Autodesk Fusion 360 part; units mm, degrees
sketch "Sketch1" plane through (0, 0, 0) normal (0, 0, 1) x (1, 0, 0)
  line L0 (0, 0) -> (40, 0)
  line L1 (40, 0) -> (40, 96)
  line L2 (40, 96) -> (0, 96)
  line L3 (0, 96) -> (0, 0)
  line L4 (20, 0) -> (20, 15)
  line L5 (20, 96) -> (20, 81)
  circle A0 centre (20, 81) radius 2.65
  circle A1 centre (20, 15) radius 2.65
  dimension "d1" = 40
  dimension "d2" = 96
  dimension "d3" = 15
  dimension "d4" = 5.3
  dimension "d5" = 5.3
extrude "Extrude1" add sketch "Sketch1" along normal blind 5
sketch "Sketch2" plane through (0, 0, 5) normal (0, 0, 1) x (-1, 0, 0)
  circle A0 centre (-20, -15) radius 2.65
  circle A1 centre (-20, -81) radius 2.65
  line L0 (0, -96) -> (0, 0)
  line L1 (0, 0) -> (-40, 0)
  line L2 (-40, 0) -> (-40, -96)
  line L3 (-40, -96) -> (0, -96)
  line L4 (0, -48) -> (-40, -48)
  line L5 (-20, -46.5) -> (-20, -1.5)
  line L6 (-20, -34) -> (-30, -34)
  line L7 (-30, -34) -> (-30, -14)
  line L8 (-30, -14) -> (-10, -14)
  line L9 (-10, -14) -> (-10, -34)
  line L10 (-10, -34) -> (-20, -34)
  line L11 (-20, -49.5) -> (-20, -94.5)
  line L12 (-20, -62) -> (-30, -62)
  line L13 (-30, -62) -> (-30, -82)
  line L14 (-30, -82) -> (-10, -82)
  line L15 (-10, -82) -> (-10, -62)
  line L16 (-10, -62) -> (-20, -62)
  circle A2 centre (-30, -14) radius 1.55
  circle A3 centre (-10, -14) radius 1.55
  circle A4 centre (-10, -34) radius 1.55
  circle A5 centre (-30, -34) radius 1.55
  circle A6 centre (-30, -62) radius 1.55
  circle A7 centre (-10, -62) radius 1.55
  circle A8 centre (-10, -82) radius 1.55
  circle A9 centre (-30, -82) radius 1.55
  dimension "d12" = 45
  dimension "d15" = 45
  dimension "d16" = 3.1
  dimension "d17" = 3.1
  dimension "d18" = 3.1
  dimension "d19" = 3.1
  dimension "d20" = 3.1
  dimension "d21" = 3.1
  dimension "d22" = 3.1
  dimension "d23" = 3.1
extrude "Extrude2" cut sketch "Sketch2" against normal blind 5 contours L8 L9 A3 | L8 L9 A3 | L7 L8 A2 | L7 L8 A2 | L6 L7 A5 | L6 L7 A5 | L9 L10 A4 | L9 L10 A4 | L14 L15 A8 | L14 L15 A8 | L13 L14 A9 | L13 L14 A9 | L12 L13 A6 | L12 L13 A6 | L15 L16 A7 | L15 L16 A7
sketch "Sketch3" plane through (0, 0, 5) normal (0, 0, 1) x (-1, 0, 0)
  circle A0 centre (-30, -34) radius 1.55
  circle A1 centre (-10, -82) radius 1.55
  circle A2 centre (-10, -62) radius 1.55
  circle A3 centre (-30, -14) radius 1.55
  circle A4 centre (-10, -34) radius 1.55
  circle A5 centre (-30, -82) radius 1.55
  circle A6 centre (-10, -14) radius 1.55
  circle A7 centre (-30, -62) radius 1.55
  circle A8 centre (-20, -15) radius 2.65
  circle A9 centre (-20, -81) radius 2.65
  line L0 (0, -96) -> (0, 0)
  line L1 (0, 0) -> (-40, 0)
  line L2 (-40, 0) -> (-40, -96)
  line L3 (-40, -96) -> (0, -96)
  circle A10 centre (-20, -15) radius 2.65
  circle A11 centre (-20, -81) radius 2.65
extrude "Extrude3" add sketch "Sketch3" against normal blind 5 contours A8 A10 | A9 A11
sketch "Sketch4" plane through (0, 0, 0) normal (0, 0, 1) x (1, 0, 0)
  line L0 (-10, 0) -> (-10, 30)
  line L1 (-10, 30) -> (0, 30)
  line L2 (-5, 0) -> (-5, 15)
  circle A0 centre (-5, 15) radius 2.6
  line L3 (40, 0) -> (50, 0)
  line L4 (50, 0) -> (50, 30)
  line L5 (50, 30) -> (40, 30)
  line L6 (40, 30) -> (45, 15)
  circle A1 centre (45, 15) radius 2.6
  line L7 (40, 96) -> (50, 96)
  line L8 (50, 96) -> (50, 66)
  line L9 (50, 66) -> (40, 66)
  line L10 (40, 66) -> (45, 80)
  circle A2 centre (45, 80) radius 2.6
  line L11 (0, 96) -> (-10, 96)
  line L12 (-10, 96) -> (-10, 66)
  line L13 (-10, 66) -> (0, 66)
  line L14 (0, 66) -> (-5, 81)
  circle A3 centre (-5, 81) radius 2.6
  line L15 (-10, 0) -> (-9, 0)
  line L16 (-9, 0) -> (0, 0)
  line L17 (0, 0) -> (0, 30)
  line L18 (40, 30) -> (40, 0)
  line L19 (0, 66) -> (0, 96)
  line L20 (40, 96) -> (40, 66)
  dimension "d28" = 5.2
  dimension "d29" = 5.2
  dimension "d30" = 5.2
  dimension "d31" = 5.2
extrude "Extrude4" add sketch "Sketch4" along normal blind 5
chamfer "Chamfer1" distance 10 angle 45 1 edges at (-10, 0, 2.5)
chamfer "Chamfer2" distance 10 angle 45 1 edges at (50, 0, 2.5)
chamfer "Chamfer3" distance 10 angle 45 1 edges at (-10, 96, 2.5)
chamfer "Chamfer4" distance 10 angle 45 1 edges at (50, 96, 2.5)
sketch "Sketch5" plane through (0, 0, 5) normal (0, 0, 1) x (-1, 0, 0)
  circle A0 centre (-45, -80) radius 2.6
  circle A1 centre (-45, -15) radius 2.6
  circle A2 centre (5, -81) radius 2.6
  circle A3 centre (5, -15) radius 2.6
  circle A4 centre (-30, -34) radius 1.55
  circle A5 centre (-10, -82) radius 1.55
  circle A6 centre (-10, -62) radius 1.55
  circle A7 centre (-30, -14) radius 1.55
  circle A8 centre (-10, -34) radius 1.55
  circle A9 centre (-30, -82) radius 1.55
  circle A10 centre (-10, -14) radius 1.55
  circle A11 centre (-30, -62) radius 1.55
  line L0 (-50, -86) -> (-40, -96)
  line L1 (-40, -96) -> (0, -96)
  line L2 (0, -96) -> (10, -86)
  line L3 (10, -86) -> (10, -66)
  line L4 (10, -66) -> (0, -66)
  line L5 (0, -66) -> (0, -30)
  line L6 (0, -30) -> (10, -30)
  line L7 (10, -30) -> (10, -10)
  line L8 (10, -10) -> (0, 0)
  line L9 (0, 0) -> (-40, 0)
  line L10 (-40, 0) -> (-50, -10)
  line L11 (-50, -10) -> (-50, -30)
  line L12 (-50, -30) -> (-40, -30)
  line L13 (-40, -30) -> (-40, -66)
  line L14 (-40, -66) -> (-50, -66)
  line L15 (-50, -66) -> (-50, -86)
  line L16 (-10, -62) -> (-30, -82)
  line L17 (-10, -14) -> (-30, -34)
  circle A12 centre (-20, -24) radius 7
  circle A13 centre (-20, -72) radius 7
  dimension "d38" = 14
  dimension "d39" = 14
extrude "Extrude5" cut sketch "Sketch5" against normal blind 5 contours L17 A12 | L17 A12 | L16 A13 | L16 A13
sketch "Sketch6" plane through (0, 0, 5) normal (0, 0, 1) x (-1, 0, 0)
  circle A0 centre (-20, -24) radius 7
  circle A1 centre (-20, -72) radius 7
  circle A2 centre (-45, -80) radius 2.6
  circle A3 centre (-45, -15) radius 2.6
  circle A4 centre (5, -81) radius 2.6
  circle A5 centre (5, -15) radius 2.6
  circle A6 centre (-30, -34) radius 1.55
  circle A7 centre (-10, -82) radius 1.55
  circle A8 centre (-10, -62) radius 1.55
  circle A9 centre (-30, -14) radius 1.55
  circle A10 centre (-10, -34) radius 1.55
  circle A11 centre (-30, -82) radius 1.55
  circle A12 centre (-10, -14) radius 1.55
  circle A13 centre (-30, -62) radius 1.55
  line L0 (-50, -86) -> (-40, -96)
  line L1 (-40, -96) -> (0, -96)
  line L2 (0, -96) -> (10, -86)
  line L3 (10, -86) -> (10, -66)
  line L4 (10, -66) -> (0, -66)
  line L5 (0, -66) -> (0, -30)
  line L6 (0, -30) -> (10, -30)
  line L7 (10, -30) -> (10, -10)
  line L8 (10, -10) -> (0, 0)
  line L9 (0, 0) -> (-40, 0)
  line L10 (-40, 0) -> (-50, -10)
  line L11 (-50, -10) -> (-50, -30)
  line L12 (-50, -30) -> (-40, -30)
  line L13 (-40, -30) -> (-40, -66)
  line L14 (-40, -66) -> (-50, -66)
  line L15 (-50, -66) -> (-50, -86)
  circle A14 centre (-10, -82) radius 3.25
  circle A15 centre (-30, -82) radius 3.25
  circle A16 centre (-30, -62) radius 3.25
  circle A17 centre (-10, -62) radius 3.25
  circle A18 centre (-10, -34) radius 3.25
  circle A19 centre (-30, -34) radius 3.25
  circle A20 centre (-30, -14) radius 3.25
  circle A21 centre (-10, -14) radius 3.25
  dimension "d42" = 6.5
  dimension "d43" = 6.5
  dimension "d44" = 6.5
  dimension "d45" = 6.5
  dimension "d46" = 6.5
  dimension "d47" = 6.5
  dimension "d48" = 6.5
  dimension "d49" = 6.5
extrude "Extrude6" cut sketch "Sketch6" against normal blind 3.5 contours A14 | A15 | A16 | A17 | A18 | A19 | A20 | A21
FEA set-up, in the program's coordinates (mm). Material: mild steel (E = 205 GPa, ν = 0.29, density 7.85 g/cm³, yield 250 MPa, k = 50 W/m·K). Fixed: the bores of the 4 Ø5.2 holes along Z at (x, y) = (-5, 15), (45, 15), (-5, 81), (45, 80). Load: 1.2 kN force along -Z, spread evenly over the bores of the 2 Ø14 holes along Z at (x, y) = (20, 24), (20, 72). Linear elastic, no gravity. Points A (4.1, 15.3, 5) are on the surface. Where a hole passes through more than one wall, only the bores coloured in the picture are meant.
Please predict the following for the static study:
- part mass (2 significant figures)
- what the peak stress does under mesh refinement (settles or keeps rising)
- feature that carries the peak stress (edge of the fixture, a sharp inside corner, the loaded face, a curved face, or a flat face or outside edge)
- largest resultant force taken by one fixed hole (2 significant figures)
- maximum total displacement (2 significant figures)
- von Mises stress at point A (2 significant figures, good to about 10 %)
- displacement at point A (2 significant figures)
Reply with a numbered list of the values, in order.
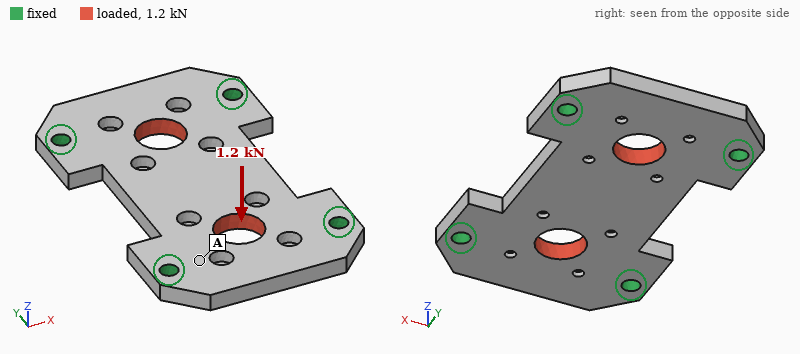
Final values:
1. 170 g
2. keeps rising
3. edge of the fixture
4. 310 N
5. 13 µm
6. 21 MPa
7. 2.6 µm
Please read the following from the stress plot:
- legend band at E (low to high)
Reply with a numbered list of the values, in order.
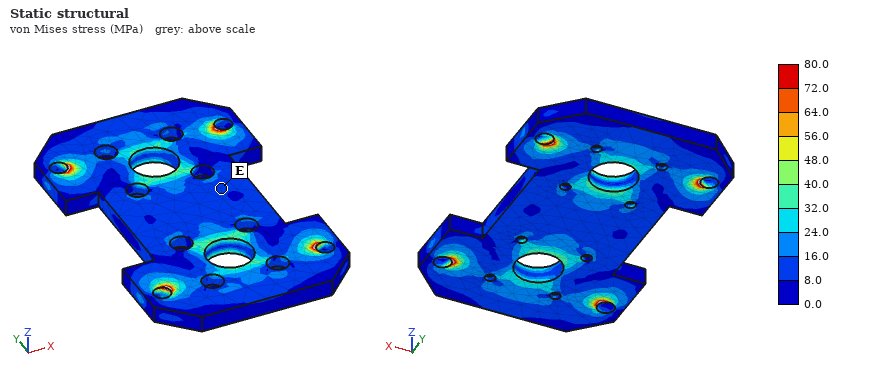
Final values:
1. 8.0 to 16.0 MPa
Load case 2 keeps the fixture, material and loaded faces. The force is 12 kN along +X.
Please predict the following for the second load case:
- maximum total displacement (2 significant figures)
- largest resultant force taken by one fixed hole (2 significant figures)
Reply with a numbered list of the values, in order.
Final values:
1. 7.0 µm
2. 3.3 kN
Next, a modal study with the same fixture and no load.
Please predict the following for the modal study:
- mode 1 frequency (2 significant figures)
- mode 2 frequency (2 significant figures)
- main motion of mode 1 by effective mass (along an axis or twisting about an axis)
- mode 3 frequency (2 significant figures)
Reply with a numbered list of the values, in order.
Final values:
1. 5000 Hz
2. 8800 Hz
3. along Z
4. 9000 Hz
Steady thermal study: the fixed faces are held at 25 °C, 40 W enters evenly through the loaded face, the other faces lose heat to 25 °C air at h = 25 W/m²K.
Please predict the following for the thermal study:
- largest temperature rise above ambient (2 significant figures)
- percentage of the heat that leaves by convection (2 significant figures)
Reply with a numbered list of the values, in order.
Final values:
1. 40 K
2. 13 %
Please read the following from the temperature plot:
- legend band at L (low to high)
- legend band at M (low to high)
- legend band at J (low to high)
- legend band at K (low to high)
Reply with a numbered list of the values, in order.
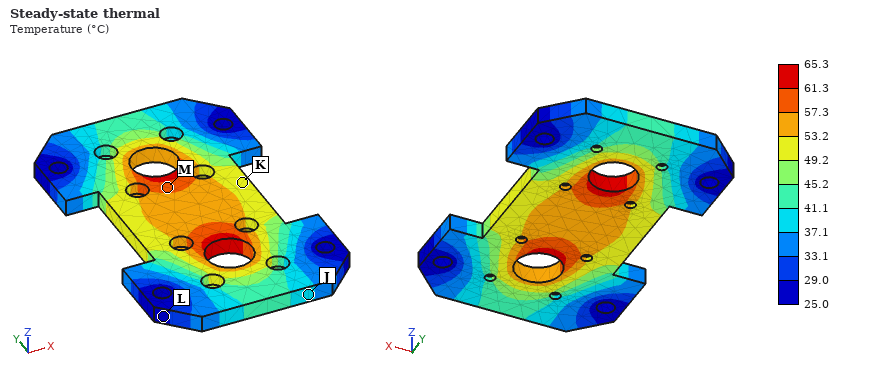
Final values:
1. 25.0 to 29.0 °C
2. 57.3 to 61.3 °C
3. 37.1 to 41.1 °C
4. 49.2 to 53.2 °C
